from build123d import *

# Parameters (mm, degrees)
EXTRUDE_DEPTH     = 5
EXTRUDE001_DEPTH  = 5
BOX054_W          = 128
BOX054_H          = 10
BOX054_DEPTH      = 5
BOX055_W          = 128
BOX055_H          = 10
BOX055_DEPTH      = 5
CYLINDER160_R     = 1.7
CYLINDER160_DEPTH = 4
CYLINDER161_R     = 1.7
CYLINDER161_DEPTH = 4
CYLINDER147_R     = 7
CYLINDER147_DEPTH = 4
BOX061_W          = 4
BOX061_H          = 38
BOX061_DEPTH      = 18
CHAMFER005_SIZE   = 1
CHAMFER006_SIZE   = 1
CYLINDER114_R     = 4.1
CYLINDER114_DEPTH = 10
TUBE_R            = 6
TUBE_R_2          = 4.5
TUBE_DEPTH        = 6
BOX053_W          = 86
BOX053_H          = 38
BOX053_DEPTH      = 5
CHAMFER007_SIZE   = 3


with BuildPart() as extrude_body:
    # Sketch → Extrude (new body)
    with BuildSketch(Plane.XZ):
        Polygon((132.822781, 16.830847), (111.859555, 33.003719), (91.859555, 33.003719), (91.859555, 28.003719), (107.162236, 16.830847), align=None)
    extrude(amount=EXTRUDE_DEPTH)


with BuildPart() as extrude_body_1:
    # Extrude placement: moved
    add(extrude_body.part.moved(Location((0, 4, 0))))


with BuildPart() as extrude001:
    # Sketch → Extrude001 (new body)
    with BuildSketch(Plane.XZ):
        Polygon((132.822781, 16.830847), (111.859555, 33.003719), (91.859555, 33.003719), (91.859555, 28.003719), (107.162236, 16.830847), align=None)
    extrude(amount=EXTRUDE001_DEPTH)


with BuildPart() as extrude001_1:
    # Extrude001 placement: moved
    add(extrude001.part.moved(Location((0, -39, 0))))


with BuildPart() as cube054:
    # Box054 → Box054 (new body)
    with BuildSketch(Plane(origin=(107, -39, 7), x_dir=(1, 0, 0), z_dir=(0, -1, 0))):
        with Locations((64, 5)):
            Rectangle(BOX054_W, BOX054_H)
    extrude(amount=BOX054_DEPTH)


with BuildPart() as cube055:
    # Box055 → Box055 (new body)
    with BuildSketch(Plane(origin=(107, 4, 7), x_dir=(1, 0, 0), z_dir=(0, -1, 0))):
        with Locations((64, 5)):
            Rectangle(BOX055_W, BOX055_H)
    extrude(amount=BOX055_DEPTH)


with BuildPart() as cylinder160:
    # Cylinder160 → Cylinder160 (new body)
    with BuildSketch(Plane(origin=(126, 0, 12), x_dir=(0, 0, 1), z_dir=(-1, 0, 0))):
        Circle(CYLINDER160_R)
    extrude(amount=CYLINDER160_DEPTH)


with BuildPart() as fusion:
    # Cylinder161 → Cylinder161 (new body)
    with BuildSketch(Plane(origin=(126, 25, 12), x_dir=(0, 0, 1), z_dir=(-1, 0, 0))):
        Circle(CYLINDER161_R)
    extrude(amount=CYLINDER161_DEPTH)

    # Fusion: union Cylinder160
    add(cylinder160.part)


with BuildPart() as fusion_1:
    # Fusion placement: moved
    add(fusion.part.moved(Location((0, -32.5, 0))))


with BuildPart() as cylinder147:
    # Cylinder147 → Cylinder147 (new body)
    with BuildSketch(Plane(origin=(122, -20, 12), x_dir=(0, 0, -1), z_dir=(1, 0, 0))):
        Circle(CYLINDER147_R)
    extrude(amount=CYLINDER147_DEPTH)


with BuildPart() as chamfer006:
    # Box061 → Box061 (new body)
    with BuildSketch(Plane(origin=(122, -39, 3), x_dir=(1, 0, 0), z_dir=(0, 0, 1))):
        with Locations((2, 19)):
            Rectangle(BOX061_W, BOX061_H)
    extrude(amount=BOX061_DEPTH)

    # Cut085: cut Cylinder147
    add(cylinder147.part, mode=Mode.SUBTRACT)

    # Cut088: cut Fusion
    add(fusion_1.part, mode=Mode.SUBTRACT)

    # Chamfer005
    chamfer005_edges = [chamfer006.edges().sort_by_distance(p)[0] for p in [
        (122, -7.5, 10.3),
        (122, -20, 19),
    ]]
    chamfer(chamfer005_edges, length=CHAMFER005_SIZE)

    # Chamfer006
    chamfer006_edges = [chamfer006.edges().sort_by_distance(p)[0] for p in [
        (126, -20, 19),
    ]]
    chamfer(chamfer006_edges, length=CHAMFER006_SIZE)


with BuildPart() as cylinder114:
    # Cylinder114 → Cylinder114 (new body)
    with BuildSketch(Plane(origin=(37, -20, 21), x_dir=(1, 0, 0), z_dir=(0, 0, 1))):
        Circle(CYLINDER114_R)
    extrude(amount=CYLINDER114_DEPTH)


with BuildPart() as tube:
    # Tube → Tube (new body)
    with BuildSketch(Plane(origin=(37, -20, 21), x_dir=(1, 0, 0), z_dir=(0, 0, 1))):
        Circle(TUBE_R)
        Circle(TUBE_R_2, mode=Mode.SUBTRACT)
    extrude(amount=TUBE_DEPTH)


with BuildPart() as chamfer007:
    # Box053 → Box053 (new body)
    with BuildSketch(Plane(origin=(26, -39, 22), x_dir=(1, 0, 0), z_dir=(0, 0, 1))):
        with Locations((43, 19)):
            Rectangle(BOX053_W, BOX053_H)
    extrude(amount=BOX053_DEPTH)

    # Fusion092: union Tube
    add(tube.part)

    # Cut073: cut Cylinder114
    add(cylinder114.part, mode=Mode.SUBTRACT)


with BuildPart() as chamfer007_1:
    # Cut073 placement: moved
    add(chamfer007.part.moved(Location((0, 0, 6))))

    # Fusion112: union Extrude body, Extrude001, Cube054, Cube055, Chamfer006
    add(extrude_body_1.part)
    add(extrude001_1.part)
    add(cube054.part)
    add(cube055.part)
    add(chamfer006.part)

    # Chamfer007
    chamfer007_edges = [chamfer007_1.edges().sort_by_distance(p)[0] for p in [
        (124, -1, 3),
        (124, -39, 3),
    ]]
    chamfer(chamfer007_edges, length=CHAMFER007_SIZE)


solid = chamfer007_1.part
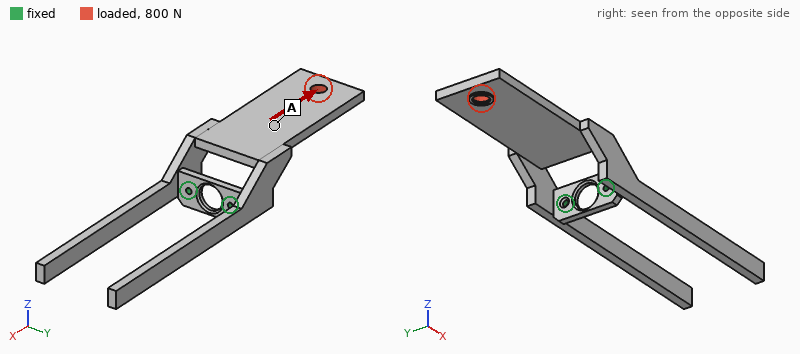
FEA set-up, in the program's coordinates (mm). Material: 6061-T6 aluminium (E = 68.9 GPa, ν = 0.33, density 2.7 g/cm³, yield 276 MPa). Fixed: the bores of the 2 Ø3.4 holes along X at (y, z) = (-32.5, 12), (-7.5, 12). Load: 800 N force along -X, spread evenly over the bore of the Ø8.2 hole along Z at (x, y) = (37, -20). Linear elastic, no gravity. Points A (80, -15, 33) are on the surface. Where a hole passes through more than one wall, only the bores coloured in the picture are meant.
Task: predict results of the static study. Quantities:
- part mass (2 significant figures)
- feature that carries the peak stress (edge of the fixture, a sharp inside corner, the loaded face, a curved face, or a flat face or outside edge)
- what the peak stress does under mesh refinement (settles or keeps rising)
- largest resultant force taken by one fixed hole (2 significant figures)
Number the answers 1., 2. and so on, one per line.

1. 94 g
2. edge of the fixture
3. keeps rising
4. 410 N
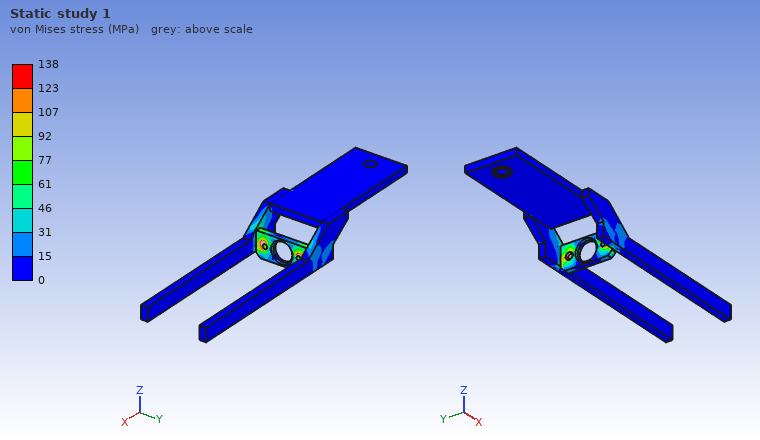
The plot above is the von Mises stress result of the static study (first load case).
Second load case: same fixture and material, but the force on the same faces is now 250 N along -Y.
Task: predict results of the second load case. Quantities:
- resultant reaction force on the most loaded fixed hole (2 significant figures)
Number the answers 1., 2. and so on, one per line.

1. 580 N
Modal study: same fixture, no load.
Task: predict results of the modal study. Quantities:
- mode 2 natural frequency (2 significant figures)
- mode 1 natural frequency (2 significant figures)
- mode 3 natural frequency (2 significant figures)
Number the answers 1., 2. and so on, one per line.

1. 320 Hz
2. 300 Hz
3. 380 Hz
